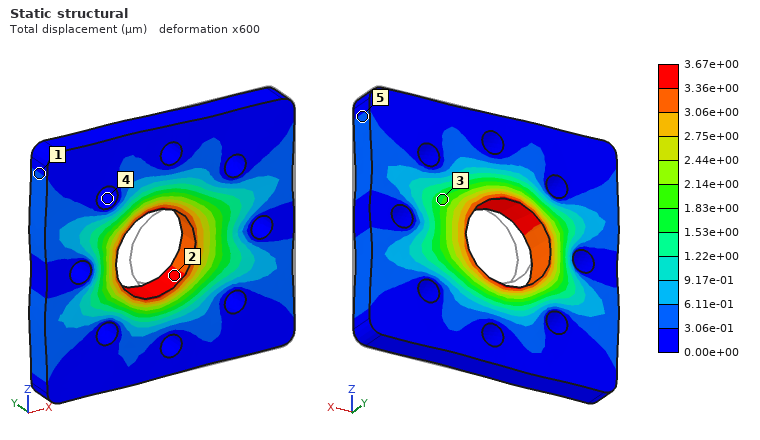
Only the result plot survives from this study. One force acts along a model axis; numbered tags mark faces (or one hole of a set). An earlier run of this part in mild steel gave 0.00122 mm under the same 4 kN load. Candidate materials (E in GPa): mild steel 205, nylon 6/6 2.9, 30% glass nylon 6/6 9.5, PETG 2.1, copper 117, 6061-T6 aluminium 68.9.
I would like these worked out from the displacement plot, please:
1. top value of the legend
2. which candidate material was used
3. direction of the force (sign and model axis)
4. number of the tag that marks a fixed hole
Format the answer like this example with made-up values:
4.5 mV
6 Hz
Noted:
3.67e+00 µm
6061-T6 aluminium
-X
4
